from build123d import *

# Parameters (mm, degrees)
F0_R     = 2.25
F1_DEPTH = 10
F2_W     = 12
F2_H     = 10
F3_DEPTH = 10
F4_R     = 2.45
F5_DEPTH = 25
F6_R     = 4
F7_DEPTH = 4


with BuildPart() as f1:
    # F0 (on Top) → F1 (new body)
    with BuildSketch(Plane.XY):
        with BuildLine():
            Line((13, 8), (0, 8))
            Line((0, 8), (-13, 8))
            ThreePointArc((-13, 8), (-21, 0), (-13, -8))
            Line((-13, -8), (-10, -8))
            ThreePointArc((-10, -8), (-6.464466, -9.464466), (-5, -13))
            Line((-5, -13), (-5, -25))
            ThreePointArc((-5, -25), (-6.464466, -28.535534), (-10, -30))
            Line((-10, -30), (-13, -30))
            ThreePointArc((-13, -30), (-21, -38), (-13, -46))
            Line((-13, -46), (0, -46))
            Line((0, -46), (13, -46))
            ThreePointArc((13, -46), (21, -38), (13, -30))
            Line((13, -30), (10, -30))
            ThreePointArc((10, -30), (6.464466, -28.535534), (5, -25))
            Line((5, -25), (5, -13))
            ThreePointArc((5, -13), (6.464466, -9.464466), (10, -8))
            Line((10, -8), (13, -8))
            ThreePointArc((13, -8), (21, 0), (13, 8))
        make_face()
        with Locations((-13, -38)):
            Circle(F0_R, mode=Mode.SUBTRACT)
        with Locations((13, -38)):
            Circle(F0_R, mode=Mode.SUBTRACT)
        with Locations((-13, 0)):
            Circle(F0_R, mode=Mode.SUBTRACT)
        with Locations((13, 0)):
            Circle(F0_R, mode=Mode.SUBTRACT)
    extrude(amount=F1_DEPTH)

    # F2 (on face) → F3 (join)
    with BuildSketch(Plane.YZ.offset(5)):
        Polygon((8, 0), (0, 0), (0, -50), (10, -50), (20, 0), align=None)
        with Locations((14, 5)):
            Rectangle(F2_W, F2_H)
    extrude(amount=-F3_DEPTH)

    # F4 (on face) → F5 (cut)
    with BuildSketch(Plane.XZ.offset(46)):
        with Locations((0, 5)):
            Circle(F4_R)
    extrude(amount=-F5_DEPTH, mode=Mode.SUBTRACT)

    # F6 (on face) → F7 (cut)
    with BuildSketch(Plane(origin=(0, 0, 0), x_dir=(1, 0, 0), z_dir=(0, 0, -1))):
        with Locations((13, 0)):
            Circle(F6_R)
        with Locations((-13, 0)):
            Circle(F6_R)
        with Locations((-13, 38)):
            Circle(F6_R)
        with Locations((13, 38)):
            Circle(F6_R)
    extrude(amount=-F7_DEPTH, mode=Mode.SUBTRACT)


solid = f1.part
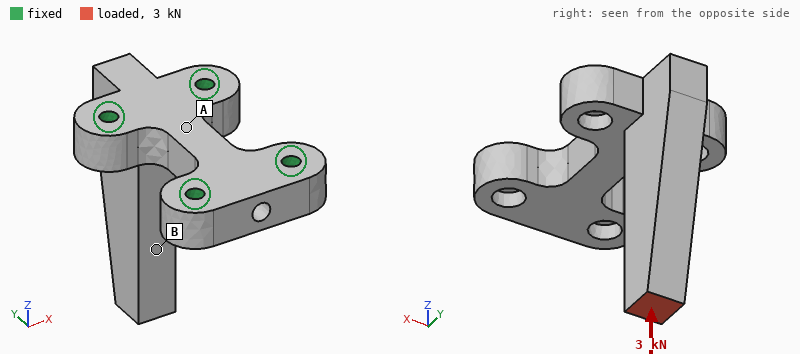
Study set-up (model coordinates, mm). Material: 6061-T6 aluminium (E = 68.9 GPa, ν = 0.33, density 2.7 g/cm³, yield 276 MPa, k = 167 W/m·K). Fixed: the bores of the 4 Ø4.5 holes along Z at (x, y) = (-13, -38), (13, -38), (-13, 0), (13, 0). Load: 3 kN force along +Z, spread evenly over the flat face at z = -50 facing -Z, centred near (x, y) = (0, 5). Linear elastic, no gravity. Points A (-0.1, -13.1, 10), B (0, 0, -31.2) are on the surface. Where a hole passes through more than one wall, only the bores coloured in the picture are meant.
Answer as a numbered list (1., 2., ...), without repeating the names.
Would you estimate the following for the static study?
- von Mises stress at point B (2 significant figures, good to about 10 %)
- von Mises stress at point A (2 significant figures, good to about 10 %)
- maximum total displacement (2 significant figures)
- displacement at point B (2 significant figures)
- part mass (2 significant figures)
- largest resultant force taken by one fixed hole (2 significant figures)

1. 39 MPa
2. 10 MPa
3. 44 µm
4. 39 µm
5. 59 g
6. 1.7 kN
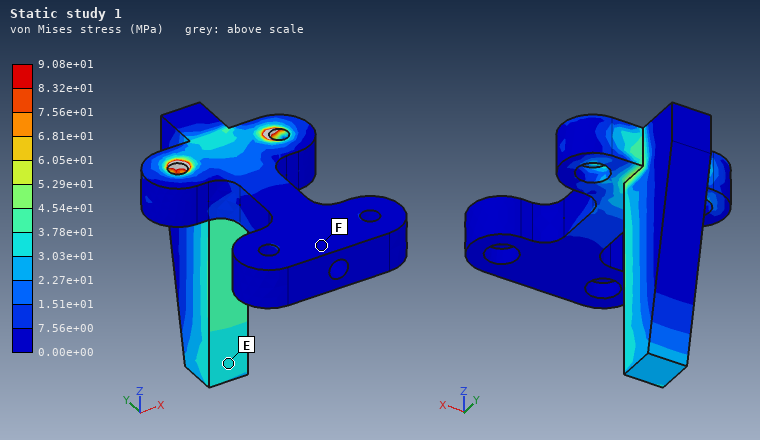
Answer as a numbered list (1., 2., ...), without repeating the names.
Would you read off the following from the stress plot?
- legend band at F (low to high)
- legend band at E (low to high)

1. 0.00e+00 to 7.56e+00 MPa
2. 3.03e+01 to 3.78e+01 MPa
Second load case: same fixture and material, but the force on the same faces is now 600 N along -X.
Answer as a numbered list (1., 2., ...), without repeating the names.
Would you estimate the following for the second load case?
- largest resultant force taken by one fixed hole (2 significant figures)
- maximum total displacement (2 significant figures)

1. 1.5 kN
2. 0.38 mm
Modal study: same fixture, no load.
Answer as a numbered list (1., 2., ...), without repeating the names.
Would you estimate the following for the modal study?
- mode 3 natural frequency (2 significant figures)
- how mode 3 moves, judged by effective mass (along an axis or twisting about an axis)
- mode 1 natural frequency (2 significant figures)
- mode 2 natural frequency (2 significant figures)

1. 12 kHz
2. along Z
3. 2900 Hz
4. 3000 Hz
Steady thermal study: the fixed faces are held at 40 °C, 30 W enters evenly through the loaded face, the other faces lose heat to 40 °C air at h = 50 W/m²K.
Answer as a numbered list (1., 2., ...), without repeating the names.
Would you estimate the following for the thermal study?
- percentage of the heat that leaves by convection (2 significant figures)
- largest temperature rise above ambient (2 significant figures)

1. 16 %
2. 69 K
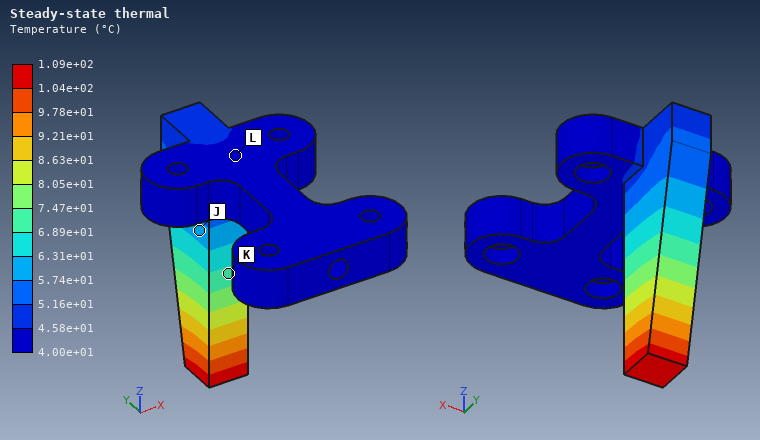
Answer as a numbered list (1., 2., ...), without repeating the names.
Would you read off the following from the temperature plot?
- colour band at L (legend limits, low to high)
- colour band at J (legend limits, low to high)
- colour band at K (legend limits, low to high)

1. 4.00e+01 to 4.58e+01 °C
2. 5.74e+01 to 6.31e+01 °C
3. 6.89e+01 to 7.47e+01 °C
